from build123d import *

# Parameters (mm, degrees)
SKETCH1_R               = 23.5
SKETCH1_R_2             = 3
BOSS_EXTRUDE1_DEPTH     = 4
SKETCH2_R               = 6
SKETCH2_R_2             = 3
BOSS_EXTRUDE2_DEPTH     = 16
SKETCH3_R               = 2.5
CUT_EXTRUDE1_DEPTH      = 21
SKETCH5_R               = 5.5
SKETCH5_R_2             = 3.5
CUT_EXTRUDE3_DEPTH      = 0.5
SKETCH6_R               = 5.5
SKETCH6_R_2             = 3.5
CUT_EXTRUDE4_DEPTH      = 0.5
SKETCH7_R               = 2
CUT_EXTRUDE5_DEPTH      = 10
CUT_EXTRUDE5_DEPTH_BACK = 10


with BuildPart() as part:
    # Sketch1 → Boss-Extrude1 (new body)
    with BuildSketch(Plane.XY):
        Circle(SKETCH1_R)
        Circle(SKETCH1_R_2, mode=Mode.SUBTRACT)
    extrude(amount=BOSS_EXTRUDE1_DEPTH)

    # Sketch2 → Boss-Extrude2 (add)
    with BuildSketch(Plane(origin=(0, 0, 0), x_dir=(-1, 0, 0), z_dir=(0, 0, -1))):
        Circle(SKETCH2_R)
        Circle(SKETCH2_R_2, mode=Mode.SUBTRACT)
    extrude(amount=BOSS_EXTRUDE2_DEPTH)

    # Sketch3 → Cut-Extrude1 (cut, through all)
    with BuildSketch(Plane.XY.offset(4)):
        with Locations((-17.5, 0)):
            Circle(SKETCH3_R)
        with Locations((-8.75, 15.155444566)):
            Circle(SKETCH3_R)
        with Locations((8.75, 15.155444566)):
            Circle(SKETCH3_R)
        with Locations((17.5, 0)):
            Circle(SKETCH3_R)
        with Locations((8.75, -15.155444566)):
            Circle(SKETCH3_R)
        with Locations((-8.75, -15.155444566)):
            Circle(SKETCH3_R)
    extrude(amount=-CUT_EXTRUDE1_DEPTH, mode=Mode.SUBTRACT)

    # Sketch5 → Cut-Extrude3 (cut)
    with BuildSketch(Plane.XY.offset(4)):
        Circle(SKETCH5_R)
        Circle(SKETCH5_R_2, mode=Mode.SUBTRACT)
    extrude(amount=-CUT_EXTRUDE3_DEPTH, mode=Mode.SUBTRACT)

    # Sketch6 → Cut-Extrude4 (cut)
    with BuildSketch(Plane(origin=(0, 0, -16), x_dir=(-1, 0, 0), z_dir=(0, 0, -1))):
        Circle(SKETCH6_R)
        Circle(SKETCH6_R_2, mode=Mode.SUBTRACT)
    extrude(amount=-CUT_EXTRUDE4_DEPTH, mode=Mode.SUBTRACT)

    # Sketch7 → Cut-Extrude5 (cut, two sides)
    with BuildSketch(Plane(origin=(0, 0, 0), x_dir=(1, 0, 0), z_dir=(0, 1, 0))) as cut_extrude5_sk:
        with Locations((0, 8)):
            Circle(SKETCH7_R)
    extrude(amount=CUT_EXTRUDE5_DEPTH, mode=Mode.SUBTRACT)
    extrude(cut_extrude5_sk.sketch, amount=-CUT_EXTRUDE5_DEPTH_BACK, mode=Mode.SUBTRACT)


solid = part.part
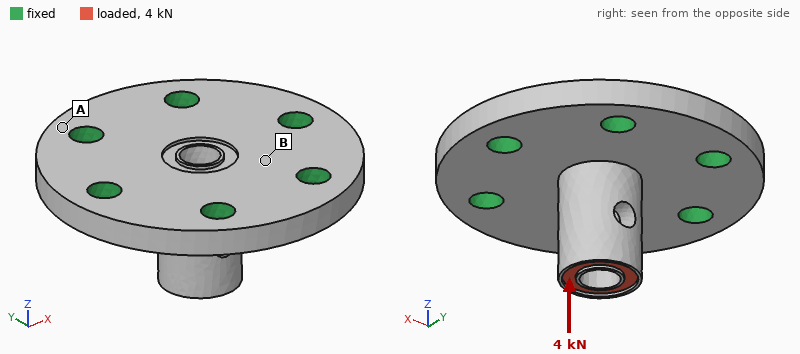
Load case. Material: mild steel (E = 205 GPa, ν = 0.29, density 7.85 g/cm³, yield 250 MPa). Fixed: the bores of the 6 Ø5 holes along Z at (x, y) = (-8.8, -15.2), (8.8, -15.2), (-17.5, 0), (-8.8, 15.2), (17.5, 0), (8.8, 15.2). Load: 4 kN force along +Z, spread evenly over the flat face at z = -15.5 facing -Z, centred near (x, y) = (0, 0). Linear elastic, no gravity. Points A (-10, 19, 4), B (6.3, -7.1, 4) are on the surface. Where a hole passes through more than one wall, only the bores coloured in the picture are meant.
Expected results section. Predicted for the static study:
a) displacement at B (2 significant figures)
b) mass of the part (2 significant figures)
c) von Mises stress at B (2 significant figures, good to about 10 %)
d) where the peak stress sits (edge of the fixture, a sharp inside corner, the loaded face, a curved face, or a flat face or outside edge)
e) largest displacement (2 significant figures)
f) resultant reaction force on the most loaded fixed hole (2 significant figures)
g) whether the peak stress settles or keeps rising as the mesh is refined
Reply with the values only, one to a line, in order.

6.5 µm
59 g
53 MPa
edge of the fixture
16 µm
730 N
keeps rising
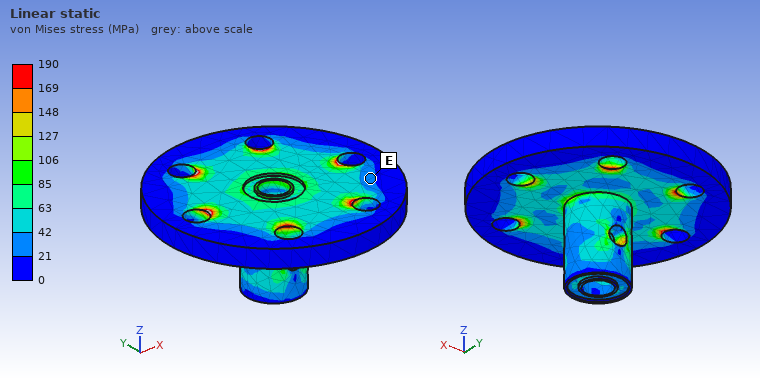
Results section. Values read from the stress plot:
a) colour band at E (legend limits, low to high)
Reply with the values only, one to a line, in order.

21 to 42 MPa
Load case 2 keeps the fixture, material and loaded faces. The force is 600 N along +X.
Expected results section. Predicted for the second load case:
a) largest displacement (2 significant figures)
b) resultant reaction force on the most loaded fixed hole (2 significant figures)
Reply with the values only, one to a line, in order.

18 µm
330 N
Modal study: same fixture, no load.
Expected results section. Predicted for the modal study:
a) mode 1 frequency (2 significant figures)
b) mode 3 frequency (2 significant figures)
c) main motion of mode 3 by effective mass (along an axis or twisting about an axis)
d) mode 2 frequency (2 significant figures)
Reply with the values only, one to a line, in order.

16 kHz
23 kHz
along Z
16 kHz
